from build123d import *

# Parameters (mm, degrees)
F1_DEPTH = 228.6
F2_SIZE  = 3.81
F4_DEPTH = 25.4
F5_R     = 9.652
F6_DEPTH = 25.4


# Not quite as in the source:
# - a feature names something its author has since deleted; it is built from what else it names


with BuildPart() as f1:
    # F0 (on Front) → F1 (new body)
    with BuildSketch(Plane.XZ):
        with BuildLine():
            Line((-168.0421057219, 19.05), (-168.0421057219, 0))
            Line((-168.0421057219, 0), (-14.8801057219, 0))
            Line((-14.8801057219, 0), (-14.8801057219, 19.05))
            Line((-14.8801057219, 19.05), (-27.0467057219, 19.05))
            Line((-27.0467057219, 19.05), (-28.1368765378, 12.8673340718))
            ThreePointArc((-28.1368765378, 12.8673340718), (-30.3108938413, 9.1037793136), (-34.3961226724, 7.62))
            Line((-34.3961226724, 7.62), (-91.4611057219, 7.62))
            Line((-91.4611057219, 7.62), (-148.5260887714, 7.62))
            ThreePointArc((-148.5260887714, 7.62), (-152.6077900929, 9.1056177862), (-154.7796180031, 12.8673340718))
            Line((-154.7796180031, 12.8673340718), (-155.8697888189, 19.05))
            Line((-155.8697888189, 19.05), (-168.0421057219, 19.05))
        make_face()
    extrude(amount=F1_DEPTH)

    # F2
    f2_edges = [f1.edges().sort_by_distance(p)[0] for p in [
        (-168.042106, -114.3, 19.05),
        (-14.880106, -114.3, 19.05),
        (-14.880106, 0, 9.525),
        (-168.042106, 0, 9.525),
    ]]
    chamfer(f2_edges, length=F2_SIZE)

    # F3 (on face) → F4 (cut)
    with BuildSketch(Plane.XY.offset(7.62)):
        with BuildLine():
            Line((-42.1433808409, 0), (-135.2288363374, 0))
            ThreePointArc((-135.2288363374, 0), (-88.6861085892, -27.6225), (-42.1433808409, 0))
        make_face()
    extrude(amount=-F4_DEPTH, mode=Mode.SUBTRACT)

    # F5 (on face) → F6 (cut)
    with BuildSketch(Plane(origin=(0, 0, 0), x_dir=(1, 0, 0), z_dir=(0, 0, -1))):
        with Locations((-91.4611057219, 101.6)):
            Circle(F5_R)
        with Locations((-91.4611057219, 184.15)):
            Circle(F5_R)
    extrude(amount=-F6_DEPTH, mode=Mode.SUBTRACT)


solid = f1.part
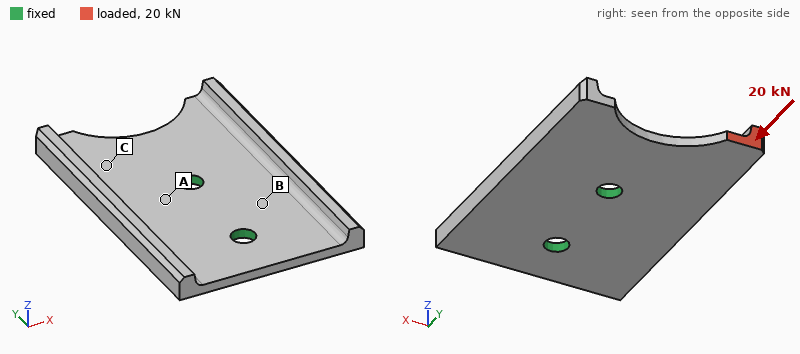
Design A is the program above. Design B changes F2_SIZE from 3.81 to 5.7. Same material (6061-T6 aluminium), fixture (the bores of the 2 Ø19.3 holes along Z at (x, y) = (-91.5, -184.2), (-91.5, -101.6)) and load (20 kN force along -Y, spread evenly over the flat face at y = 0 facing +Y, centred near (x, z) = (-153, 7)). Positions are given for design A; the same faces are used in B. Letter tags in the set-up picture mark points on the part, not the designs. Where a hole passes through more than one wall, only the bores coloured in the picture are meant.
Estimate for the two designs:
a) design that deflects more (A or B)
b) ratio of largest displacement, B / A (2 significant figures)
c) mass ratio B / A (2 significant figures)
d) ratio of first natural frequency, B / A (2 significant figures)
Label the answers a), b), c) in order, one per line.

a) A
b) 0.92
c) 0.99
d) 1.0
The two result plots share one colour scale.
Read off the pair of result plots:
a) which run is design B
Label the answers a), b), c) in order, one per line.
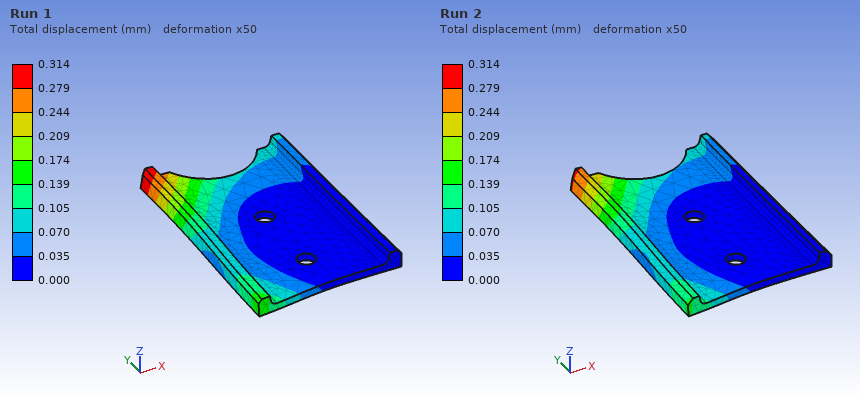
a) Run 2
